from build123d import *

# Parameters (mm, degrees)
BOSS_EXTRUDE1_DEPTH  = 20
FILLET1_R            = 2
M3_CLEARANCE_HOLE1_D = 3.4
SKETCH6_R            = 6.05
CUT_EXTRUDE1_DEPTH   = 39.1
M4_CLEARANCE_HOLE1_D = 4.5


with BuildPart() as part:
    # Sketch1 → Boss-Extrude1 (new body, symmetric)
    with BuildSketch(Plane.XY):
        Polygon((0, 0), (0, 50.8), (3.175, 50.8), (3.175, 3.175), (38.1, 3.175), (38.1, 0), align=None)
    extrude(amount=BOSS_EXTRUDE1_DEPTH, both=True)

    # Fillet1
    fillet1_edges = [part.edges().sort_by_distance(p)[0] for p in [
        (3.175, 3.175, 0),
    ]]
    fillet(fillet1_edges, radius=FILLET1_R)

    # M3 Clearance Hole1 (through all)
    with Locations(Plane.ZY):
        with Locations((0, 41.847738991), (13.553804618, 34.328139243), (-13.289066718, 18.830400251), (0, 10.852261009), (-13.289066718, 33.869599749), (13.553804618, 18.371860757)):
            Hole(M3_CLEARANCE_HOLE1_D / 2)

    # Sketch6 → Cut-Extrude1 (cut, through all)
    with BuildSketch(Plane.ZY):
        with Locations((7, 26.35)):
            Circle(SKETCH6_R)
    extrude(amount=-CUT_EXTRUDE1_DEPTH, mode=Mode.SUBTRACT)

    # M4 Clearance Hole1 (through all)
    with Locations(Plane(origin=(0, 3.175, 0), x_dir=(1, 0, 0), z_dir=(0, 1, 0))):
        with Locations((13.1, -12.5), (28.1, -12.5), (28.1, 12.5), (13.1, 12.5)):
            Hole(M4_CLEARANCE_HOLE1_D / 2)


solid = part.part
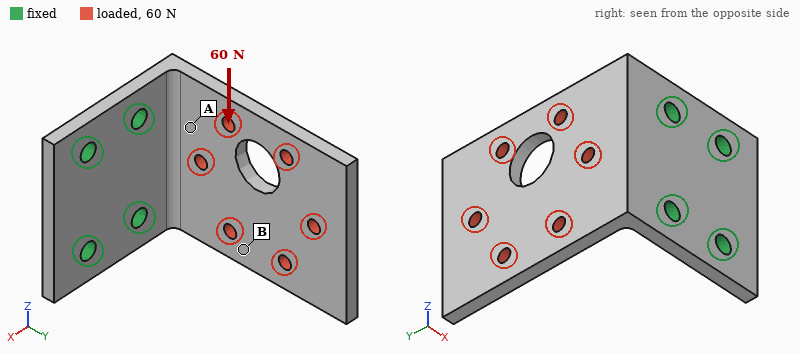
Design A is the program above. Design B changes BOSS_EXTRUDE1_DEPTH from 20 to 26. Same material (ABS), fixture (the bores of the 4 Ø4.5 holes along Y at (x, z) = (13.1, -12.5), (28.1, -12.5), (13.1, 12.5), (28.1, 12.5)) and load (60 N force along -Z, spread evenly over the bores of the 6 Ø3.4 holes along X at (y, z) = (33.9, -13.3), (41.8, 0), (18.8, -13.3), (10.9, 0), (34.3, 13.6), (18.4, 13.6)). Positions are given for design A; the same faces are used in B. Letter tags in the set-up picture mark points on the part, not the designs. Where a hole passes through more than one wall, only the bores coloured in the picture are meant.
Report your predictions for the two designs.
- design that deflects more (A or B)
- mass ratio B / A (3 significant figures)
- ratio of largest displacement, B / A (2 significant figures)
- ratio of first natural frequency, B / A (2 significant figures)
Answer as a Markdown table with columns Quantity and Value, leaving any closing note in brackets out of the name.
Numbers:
| Quantity | Value |
|---|---|
| design that deflects more | A |
| mass ratio B / A | 1.32 |
| ratio of largest displacement, B / A | 0.86 |
| ratio of first natural frequency, B / A | 0.99 |
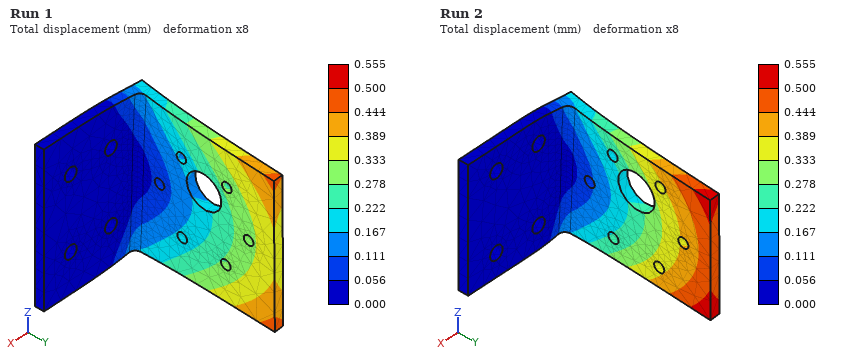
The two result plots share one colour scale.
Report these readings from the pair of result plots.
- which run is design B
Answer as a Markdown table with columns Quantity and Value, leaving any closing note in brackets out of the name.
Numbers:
| Quantity | Value |
|---|---|
| which run is design B | Run 1 |
